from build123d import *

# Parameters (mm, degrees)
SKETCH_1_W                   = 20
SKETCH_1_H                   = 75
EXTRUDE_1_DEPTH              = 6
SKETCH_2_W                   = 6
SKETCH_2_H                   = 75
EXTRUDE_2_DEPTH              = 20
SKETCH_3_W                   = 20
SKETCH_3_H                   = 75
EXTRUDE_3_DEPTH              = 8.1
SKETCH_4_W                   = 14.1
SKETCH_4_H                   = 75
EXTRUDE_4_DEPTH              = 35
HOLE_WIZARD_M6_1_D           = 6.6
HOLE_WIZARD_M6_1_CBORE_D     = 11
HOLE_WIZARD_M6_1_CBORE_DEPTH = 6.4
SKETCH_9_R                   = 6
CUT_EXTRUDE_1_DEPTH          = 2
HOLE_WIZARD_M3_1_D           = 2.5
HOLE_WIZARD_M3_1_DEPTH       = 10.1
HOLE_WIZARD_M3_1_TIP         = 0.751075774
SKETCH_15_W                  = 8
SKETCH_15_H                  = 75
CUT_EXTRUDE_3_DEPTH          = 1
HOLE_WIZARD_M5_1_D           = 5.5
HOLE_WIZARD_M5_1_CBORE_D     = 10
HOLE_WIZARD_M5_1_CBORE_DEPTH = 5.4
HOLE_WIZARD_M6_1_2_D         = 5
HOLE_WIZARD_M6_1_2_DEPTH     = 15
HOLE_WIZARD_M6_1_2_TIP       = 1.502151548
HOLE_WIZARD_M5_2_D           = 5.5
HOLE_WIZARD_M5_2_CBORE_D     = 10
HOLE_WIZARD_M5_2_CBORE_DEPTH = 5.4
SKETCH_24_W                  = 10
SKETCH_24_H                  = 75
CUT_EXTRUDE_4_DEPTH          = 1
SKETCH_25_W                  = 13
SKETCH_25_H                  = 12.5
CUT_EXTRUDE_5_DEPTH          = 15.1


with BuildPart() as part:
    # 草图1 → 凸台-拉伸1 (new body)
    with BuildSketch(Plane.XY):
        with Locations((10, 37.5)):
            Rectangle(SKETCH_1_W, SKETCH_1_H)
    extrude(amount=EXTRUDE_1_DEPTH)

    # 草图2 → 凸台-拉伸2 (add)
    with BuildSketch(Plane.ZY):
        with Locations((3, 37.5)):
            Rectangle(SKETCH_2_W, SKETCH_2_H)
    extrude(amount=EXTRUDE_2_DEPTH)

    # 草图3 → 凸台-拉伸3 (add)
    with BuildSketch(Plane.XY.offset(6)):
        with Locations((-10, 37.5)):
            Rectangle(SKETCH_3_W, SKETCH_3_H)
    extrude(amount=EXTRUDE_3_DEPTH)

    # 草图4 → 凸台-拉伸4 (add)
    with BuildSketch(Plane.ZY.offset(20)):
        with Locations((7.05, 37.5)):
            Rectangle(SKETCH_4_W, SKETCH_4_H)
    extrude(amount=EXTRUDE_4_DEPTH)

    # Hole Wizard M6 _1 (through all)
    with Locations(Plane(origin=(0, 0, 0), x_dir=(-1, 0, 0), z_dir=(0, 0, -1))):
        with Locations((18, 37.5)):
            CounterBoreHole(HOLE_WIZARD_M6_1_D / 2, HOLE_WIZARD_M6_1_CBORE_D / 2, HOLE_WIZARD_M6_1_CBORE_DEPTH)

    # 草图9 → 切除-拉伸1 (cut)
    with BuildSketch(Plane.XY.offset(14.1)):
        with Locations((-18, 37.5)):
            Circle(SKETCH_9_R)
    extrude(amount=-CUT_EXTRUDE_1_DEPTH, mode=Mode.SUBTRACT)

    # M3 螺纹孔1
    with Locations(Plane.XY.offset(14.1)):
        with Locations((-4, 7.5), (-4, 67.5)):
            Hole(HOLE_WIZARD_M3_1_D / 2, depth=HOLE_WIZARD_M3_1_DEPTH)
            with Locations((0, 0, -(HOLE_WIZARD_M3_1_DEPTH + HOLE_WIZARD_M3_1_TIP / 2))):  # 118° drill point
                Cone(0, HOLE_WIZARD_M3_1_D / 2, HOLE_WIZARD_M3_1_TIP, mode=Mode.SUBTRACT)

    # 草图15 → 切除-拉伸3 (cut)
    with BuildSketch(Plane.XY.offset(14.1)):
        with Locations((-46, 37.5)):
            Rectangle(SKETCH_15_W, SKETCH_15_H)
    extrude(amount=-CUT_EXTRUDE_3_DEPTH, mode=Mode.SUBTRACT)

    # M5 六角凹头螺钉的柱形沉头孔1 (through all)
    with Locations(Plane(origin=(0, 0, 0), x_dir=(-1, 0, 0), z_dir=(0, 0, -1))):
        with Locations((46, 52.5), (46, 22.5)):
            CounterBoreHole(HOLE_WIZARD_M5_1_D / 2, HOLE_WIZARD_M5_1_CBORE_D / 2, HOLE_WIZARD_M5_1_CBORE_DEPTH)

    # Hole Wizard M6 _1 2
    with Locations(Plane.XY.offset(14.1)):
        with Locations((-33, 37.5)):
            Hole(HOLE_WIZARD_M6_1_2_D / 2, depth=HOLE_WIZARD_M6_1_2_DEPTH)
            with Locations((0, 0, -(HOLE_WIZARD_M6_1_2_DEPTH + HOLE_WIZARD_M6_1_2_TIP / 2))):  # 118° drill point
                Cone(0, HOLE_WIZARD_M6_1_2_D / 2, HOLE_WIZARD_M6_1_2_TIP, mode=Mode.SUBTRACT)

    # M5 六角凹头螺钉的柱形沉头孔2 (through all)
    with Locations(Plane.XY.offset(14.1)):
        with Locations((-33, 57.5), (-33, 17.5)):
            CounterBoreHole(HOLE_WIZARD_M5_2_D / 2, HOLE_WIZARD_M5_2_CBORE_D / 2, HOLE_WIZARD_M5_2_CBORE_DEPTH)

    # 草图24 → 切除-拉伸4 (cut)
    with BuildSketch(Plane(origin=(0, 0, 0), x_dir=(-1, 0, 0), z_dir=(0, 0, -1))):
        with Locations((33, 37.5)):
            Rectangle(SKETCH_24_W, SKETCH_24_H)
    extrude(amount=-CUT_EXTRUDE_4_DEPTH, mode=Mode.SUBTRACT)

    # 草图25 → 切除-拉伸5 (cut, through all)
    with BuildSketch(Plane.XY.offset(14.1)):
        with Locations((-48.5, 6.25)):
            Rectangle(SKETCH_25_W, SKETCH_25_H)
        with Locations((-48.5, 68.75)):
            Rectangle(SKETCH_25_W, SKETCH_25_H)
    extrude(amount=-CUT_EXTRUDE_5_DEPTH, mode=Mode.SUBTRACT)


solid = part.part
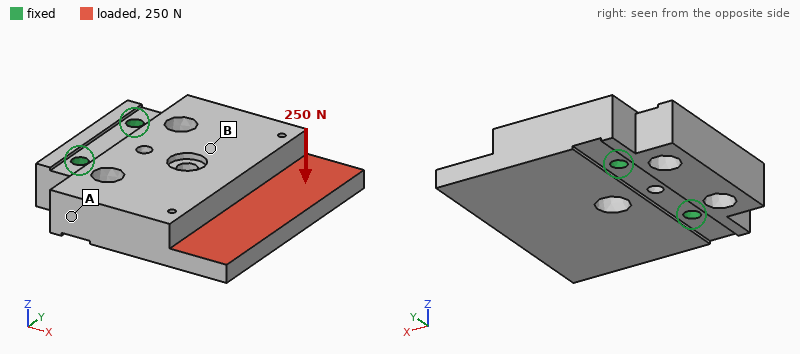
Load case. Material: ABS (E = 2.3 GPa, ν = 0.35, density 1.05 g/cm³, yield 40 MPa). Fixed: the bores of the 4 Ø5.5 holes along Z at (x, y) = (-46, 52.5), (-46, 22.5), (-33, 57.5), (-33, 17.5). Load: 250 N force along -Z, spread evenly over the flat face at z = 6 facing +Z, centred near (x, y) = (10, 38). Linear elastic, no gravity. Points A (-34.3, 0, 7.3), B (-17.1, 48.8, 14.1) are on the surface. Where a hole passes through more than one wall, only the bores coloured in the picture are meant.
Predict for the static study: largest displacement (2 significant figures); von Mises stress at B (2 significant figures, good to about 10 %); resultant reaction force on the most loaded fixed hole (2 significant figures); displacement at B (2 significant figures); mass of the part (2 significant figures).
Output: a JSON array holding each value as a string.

["0.59 mm", "3.4 MPa", "330 N", "0.12 mm", "60 g"]
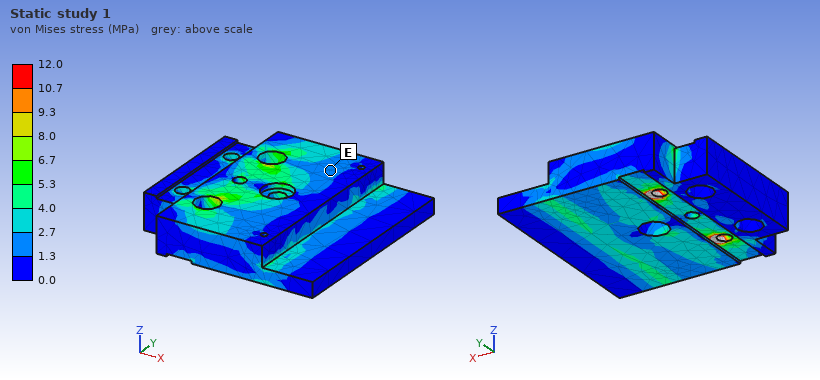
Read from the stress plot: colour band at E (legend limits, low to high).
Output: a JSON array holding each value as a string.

["1.3 to 2.7 MPa"]
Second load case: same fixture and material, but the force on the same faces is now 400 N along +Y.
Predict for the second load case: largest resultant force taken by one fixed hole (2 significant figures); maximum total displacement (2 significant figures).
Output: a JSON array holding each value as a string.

["390 N", "0.11 mm"]
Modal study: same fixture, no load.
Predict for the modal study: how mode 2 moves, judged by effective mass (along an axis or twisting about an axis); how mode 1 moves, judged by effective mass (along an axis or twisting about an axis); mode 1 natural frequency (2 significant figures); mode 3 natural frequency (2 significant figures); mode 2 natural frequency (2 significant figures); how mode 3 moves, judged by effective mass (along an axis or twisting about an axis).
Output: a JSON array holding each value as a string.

["twisting about X", "along Z", "1000 Hz", "2800 Hz", "1700 Hz", "along Y"]
